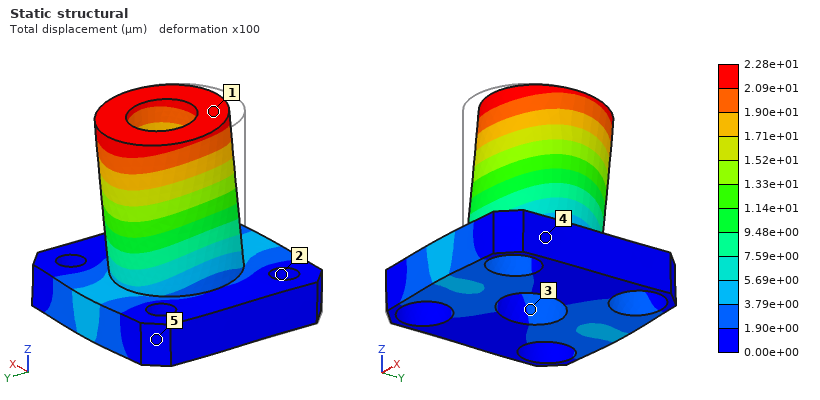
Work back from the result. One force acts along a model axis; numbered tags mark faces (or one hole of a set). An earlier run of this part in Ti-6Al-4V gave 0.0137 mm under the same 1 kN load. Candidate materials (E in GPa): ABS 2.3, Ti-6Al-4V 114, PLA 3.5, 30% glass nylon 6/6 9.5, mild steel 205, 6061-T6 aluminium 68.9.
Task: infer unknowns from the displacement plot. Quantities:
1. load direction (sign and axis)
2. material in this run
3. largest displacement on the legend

+Y
6061-T6 aluminium
2.28e+01 µm
